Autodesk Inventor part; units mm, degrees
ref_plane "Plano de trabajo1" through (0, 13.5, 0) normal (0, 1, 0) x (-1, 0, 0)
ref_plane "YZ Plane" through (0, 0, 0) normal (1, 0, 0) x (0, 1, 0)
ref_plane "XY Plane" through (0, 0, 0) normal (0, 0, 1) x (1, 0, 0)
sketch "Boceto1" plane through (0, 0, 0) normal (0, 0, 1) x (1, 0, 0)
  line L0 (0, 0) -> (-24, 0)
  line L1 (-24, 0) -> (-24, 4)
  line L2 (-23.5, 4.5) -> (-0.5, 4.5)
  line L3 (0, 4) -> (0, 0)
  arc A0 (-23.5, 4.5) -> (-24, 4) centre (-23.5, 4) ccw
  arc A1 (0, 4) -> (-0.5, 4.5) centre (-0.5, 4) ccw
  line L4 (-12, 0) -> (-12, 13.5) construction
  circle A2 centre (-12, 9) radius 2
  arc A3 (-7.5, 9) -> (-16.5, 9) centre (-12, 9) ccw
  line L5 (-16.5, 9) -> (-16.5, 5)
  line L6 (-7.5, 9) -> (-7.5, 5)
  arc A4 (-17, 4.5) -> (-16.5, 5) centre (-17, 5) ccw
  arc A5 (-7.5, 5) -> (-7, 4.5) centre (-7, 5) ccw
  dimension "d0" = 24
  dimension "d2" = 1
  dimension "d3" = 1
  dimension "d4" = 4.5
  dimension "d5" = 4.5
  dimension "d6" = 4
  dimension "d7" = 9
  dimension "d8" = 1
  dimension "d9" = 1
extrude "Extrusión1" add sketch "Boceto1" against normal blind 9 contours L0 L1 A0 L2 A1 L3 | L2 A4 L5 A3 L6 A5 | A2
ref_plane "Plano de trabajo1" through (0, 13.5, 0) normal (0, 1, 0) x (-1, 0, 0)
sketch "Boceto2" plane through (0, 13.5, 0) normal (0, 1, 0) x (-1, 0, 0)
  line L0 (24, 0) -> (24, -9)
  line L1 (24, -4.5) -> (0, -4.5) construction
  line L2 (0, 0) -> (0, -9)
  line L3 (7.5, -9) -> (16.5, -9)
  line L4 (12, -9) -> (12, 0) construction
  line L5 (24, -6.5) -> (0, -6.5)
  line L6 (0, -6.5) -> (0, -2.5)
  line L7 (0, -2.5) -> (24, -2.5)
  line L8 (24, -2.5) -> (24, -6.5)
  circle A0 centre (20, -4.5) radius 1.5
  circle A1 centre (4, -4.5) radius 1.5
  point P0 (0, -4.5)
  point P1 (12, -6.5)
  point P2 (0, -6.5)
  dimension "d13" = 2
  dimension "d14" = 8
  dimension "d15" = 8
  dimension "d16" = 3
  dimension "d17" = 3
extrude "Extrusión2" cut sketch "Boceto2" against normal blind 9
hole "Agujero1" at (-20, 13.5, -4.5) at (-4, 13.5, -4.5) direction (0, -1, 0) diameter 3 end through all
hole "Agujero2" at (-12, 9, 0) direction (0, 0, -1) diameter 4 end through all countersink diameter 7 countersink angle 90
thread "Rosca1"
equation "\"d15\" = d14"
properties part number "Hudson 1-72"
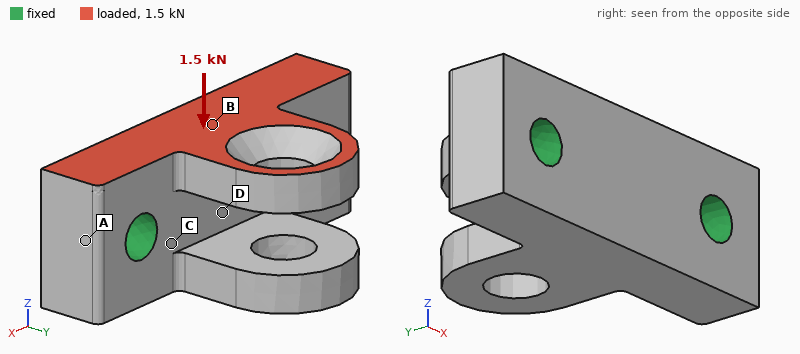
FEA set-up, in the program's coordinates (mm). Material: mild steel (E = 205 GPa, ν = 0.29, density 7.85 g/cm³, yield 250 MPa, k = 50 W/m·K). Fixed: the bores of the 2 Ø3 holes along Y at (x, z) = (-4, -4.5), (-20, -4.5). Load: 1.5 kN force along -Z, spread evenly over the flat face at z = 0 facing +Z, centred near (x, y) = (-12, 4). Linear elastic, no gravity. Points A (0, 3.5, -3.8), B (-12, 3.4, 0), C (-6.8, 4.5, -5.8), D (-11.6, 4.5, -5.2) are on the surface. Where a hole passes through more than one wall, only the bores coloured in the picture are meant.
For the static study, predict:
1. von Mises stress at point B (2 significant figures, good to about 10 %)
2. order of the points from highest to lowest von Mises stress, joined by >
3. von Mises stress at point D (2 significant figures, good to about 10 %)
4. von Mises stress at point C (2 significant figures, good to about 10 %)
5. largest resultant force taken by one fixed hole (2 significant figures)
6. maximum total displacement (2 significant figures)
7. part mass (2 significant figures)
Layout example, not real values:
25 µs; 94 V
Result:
72 MPa; B > C > D > A; 25 MPa; 45 MPa; 750 N; 31 µm; 9.3 g
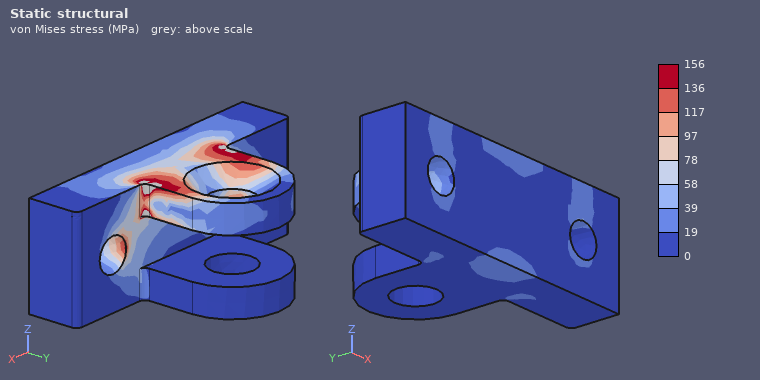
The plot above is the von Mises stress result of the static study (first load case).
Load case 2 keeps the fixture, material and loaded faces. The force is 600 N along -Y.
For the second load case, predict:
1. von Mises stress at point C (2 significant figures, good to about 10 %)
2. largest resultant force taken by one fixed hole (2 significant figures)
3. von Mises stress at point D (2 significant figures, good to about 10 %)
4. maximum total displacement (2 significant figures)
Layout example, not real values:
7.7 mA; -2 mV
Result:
19 MPa; 300 N; 11 MPa; 8.1 µm
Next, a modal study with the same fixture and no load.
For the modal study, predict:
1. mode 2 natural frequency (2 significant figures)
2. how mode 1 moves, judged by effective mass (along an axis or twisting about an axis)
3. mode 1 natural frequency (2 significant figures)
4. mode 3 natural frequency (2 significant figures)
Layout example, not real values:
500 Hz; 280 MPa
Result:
22 kHz; along Z; 20 kHz; 43 kHz
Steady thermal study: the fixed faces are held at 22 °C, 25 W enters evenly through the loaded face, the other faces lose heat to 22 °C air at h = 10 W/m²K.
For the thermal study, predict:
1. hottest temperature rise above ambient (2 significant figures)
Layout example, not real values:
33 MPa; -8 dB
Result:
66 K
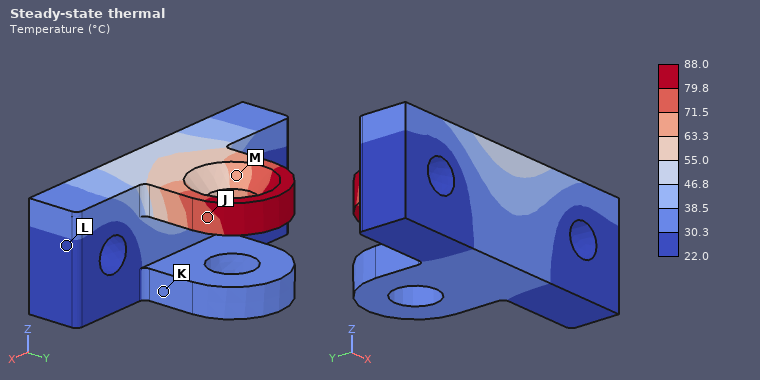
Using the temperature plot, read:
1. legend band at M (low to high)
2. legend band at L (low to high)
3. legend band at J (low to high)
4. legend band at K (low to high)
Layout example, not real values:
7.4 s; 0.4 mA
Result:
63.3 to 71.5 °C; 22.0 to 30.3 °C; 71.5 to 79.8 °C; 30.3 to 38.5 °C
